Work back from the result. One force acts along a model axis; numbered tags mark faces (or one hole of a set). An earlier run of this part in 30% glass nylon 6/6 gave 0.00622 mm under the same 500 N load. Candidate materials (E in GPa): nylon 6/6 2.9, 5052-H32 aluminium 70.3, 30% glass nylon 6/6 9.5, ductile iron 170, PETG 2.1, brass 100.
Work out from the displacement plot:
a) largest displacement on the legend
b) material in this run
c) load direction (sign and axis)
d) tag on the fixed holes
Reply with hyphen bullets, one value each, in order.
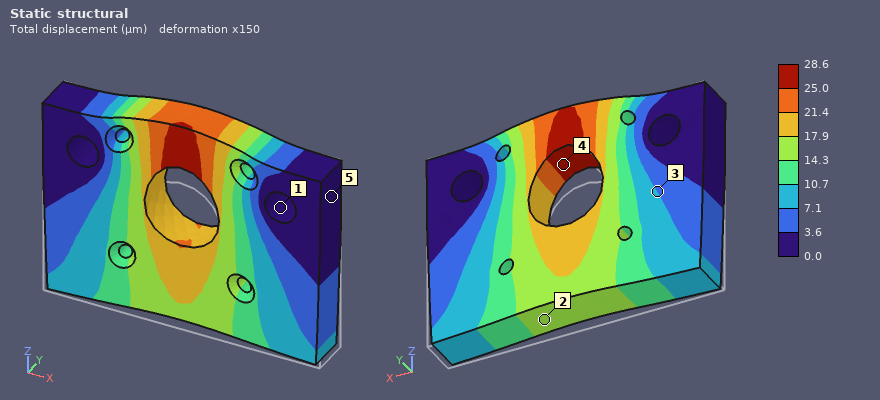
- 28.6 µm
- PETG
- +Z
- 1
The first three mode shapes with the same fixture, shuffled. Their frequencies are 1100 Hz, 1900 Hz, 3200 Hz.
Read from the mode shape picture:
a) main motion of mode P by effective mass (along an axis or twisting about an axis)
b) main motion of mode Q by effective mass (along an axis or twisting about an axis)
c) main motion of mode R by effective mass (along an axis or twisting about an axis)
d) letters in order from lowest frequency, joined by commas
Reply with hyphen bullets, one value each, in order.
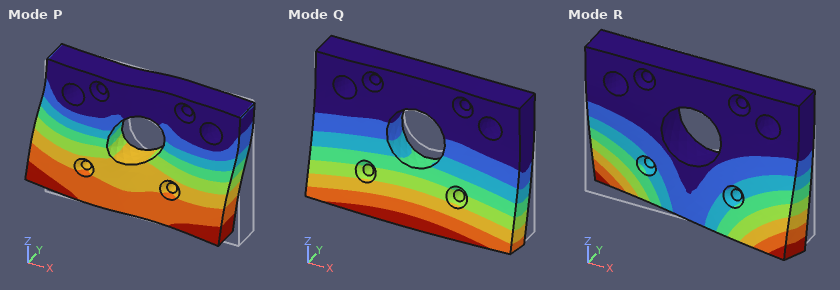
- along X
- along Y
- twisting about Z
- Q, R, P
